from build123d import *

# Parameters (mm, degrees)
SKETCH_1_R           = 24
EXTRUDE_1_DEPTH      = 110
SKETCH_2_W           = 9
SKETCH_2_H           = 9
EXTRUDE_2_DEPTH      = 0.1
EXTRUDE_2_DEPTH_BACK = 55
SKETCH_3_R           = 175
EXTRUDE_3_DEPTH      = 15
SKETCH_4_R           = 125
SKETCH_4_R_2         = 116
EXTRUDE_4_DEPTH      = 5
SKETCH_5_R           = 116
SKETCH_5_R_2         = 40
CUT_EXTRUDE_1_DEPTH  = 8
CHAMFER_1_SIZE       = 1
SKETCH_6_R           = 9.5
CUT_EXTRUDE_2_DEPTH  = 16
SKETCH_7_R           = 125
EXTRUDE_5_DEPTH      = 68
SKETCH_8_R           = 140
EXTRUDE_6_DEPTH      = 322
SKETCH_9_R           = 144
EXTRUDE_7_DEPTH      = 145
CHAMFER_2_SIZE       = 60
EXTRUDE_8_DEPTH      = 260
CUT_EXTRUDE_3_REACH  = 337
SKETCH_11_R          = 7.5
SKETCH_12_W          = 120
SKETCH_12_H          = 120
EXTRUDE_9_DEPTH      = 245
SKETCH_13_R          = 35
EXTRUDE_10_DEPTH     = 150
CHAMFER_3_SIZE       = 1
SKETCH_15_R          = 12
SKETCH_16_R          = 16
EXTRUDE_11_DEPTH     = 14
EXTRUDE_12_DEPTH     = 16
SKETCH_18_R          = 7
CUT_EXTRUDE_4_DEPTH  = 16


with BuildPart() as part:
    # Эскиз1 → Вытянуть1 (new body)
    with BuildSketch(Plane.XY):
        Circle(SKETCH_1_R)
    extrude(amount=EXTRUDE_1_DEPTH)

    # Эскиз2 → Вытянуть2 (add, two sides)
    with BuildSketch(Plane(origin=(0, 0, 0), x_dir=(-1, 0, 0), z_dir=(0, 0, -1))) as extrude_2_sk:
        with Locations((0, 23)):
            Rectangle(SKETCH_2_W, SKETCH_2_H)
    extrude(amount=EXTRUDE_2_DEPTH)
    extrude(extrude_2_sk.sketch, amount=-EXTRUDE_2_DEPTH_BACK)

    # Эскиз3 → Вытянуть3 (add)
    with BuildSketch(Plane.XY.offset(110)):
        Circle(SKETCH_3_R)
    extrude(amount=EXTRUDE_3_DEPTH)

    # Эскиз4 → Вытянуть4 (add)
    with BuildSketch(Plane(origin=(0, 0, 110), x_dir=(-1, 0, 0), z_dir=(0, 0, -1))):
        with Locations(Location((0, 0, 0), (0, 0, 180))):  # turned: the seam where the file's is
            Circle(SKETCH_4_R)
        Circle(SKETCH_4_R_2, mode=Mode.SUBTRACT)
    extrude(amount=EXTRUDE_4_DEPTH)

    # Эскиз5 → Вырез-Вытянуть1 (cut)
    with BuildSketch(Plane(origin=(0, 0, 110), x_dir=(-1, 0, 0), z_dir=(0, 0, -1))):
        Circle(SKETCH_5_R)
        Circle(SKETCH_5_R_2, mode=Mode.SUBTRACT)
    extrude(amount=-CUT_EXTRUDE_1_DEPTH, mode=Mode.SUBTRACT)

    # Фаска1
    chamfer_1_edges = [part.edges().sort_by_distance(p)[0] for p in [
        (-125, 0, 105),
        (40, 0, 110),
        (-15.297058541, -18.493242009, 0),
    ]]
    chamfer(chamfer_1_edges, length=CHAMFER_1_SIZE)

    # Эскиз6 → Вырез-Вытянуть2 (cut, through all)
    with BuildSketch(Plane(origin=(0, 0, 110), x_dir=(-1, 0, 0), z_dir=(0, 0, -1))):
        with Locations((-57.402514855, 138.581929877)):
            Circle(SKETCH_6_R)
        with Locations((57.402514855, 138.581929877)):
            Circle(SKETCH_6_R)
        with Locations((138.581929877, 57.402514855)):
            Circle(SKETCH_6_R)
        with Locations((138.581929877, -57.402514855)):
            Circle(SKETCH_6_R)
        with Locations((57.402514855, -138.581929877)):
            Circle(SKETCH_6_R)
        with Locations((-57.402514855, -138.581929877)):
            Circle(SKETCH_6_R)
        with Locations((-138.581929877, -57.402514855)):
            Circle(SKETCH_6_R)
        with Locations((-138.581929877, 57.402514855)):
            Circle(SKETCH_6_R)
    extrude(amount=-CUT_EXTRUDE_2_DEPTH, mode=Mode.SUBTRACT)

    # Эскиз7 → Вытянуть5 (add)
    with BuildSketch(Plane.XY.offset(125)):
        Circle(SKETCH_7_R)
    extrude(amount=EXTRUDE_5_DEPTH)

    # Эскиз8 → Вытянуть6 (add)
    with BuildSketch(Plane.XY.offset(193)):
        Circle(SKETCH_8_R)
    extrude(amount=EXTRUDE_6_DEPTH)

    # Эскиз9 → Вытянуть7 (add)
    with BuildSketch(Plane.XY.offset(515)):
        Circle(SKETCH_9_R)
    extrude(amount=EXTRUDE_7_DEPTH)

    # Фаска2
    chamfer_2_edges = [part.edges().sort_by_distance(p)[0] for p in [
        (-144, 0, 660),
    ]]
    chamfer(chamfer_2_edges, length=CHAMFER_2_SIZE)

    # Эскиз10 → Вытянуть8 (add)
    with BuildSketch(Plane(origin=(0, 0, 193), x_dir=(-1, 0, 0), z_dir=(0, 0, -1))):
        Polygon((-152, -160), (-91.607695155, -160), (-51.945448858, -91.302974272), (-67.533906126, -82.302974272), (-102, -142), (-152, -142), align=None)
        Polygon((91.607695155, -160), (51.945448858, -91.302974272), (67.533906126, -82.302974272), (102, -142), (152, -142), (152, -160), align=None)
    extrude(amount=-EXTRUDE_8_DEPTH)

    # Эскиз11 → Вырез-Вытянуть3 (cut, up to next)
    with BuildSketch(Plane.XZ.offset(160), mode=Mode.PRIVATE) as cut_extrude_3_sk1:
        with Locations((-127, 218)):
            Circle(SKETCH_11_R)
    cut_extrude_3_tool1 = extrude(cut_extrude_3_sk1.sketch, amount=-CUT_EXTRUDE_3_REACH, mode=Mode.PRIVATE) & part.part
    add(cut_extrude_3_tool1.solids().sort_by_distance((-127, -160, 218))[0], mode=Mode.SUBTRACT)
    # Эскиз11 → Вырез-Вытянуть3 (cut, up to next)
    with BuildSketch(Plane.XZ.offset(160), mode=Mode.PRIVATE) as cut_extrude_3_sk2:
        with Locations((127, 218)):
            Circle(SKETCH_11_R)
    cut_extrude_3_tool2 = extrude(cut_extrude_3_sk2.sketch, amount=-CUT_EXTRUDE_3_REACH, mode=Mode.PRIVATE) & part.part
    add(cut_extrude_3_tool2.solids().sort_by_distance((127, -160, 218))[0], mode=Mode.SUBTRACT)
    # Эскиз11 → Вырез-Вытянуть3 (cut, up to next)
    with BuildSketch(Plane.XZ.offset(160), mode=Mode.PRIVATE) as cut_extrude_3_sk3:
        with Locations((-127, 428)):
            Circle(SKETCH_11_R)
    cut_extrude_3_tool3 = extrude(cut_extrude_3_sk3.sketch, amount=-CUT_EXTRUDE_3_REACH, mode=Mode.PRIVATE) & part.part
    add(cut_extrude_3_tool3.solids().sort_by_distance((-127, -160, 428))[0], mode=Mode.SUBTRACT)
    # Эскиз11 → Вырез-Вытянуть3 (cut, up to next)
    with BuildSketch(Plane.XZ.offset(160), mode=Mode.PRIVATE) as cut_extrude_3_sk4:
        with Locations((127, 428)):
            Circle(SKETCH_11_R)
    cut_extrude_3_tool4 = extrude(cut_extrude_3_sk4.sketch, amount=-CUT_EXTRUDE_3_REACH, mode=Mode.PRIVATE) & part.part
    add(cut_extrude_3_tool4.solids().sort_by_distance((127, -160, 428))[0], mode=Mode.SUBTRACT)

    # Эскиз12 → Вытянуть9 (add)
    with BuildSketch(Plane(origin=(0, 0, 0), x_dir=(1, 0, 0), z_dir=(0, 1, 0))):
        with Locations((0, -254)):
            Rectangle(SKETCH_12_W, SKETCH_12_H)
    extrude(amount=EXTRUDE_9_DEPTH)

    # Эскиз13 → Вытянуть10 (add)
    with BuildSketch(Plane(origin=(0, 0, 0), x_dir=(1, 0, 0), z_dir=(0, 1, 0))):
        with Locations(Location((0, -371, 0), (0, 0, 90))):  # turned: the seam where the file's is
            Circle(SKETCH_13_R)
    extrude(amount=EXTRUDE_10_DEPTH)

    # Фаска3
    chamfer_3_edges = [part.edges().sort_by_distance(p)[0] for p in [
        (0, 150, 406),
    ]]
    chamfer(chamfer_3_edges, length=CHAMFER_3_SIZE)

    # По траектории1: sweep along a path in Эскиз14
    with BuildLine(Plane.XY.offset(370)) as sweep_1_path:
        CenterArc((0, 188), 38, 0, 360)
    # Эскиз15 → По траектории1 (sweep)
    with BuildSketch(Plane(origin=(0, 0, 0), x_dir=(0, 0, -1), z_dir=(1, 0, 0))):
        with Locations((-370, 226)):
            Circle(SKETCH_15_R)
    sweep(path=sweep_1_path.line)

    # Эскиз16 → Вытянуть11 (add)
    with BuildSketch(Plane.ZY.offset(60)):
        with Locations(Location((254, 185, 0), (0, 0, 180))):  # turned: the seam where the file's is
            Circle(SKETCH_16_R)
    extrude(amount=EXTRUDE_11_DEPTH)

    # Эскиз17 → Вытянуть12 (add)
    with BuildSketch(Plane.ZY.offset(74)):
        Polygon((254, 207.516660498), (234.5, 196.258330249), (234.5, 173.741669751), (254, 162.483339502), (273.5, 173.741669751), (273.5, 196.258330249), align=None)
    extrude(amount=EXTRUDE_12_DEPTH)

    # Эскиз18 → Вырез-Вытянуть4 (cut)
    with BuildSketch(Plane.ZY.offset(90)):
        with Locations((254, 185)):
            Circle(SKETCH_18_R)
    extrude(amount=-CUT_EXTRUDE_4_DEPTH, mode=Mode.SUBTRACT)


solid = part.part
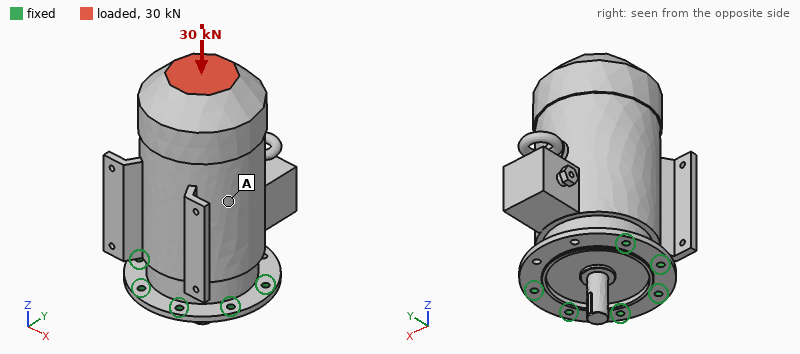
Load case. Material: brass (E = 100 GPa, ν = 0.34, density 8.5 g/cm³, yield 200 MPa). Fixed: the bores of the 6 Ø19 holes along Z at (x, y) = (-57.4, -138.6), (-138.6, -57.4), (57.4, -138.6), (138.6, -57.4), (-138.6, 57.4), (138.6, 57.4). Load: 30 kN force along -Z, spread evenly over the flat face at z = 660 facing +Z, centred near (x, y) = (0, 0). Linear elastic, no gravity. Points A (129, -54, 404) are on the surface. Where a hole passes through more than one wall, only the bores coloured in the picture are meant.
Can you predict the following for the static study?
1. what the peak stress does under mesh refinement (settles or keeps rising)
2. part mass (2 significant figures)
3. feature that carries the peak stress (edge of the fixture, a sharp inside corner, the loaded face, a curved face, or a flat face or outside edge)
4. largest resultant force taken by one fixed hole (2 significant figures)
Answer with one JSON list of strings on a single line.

["keeps rising", "300 kg", "edge of the fixture", "10 kN"]
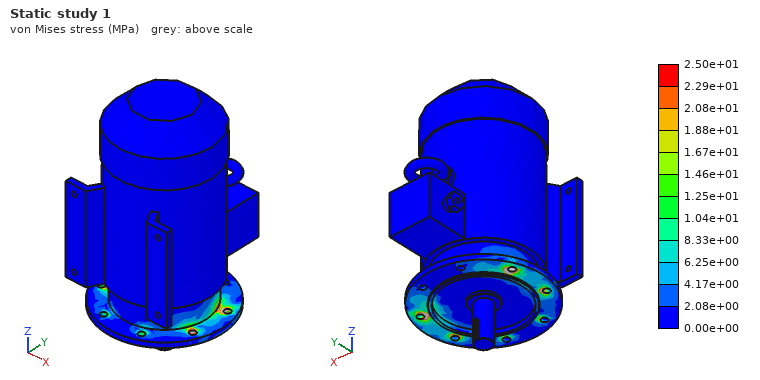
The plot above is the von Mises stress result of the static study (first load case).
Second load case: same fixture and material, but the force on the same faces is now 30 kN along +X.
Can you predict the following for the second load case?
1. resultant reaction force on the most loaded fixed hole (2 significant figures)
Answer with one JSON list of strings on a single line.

["32 kN"]
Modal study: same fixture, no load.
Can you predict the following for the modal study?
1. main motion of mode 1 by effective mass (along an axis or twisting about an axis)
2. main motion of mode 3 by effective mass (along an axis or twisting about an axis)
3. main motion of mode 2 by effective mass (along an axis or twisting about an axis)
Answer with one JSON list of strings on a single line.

["along Y", "along Z", "along X"]
